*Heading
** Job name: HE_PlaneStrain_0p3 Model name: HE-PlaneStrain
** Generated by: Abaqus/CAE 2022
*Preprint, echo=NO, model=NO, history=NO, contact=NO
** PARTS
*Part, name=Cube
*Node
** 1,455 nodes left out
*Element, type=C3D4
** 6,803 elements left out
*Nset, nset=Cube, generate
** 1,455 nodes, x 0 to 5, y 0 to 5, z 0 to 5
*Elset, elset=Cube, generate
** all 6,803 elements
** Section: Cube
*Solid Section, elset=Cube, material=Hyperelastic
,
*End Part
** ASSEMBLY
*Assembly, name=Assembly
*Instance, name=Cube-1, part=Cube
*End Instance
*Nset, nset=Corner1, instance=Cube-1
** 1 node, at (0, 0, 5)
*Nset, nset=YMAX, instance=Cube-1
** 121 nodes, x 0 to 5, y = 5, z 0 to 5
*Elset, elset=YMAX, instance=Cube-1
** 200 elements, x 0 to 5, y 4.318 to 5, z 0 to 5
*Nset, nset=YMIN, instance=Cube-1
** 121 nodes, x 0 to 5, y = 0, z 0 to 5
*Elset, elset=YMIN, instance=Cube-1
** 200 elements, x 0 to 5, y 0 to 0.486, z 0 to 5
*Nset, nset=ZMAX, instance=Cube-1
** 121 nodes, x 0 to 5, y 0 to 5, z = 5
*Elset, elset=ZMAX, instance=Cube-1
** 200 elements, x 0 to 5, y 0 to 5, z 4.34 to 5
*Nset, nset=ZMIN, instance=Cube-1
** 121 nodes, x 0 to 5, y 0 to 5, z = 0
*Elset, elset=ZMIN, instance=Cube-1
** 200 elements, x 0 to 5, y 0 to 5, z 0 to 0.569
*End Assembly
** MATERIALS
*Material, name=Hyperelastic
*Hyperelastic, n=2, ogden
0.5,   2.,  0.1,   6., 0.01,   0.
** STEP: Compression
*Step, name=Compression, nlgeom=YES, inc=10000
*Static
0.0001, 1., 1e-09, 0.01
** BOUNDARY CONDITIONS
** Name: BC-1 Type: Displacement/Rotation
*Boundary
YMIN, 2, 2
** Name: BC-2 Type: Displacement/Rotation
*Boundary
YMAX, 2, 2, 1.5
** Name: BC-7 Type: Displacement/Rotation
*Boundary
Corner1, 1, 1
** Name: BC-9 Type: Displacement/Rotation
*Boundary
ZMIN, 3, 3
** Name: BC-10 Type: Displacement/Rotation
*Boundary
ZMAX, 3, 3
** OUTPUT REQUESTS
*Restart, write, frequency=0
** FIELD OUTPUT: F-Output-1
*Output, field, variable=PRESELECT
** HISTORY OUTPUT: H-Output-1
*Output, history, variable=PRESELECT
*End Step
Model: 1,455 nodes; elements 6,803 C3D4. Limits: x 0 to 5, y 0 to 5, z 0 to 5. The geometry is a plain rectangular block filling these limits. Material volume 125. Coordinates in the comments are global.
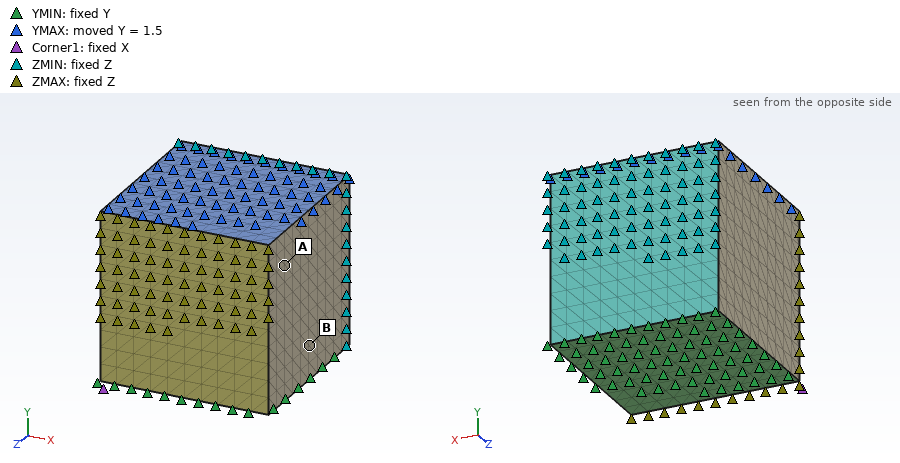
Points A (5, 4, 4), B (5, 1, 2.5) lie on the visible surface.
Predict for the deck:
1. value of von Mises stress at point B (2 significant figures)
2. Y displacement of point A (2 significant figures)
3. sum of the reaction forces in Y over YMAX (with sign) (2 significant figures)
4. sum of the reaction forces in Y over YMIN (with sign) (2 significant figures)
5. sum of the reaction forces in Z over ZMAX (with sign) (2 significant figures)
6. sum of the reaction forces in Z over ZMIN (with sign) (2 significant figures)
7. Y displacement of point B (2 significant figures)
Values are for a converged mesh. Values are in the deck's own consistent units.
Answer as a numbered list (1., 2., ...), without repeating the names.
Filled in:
1. 0.47
2. 1.2
3. 10
4. -10
5. 4.9
6. -4.9
7. 0.30
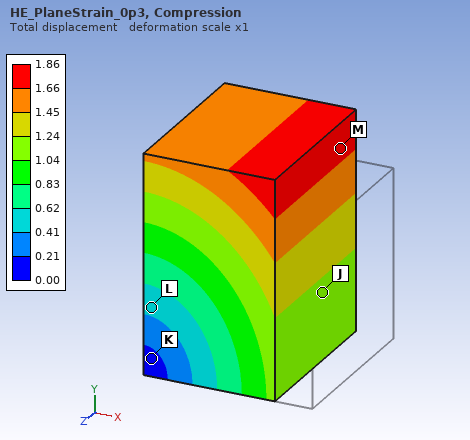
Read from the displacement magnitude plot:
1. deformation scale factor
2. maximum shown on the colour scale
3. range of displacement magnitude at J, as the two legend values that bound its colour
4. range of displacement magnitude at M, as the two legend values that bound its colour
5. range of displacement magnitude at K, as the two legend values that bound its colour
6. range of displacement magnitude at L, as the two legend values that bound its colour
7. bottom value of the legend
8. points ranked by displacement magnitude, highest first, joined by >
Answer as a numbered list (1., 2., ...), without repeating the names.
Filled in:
1. 1
2. 1.86
3. 1.04 to 1.24
4. 1.66 to 1.86
5. 0.00 to 0.21
6. 0.41 to 0.62
7. 0.00
8. M > J > L > K
